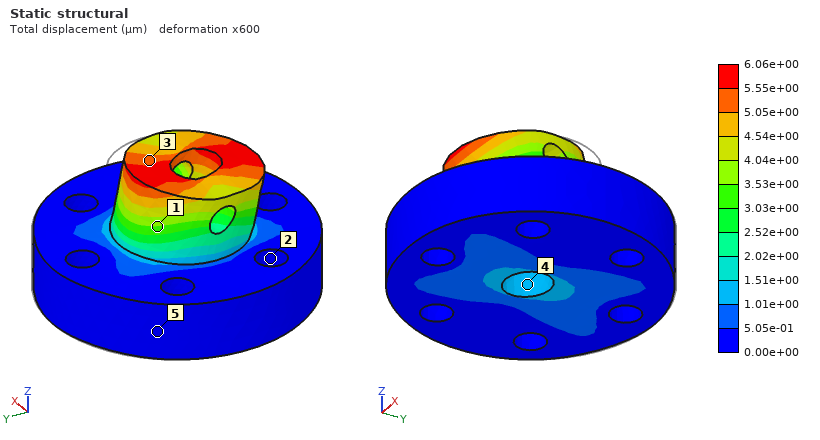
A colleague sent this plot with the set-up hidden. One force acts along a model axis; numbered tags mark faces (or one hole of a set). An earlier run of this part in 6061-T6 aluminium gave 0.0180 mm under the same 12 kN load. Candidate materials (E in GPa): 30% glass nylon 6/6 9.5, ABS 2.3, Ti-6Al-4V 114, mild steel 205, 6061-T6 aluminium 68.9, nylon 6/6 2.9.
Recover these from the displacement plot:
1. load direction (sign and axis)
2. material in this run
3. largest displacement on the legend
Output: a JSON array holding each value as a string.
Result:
["-Y", "mild steel", "6.06e+00 µm"]
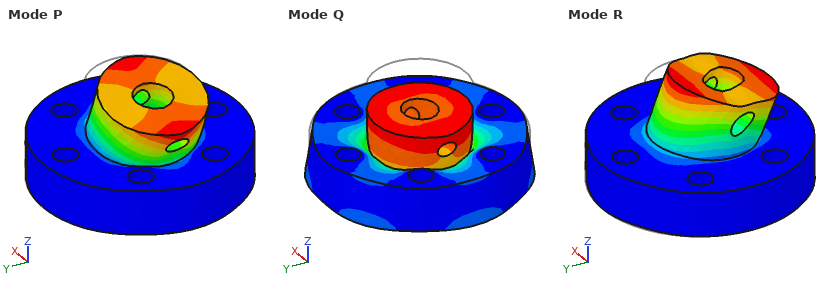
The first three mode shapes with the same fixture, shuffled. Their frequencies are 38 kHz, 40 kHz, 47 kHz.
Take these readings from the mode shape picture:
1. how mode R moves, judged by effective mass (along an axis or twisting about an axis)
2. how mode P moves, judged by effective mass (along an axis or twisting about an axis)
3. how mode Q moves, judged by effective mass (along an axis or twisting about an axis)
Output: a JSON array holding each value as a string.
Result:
["along Y", "along X", "along Z"]
